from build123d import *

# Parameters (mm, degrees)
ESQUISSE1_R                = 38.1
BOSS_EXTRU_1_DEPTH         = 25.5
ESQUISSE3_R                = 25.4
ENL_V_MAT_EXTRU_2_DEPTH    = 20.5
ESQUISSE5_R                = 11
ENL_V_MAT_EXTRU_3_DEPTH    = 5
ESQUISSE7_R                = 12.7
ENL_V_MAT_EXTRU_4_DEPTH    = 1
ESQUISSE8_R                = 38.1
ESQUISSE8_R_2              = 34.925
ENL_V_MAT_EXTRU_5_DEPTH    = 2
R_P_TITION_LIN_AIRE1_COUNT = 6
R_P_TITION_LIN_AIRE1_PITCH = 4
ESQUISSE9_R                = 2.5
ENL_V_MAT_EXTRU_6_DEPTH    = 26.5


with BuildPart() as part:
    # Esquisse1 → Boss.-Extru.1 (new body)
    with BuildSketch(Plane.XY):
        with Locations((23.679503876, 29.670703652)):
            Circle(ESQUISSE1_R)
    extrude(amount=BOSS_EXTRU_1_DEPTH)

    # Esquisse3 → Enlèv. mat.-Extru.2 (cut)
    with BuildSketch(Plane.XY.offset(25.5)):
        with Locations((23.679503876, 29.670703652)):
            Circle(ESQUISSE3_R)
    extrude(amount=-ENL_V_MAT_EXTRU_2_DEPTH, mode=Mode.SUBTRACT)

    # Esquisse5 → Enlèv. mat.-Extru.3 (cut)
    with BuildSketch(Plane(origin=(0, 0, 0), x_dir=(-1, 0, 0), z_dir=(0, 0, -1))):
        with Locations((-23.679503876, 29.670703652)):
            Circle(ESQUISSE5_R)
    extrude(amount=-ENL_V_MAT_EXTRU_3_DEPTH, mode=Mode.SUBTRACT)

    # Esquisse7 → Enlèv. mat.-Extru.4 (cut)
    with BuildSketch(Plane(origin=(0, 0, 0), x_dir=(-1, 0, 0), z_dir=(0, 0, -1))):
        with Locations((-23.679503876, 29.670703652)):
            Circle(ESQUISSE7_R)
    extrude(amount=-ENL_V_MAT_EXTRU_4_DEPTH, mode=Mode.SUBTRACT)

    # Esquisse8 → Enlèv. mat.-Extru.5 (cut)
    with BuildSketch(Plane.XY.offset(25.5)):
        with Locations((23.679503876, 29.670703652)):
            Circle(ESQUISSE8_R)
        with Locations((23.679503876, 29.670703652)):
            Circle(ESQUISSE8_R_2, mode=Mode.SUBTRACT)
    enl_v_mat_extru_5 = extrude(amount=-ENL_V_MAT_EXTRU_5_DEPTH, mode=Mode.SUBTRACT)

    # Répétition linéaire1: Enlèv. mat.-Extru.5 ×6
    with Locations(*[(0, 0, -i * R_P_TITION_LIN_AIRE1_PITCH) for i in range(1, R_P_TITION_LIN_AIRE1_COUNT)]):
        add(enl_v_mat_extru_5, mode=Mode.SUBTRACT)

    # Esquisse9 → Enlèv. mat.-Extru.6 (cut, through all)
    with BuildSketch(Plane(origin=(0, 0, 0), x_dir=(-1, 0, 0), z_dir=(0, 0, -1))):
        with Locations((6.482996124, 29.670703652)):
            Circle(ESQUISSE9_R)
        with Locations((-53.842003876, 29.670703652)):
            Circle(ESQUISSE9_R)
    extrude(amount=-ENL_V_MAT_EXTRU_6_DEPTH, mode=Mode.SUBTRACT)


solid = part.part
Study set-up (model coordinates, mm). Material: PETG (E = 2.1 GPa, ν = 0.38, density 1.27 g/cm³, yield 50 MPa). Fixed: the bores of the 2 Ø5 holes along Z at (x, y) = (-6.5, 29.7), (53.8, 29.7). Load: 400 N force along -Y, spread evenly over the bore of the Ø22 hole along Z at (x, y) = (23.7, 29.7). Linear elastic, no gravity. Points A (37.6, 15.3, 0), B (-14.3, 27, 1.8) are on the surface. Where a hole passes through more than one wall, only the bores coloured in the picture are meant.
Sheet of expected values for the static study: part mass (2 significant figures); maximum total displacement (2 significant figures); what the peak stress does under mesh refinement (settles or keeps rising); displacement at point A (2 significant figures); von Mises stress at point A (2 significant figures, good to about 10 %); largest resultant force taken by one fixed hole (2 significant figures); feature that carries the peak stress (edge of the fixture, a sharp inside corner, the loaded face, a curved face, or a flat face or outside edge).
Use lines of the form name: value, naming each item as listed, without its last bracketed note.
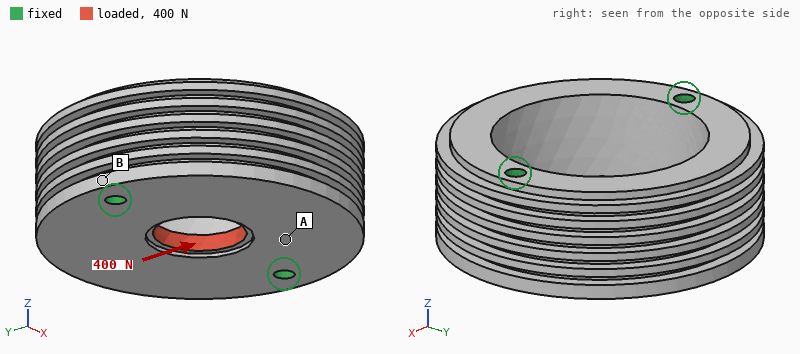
part mass: 80 g
maximum total displacement: 28 µm
what the peak stress does under mesh refinement: keeps rising
displacement at point A: 18 µm
von Mises stress at point A: 0.88 MPa
largest resultant force taken by one fixed hole: 200 N
feature that carries the peak stress: edge of the fixture
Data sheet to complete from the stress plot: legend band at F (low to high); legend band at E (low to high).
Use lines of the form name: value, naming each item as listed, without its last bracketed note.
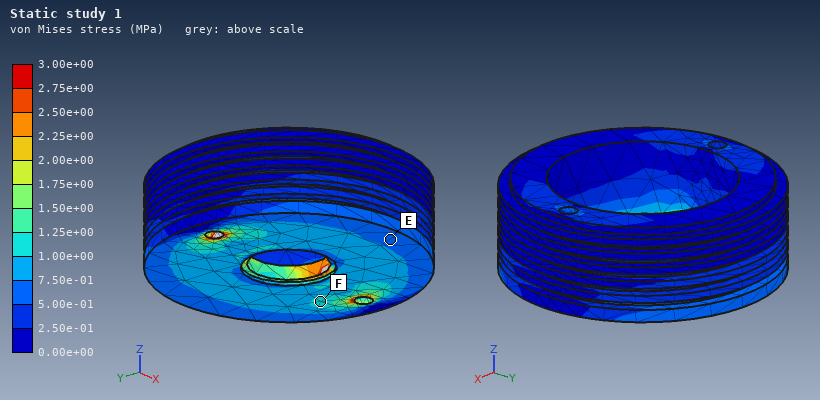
legend band at F: 1.00e+00 to 1.25e+00 MPa
legend band at E: 5.00e-01 to 7.50e-01 MPa
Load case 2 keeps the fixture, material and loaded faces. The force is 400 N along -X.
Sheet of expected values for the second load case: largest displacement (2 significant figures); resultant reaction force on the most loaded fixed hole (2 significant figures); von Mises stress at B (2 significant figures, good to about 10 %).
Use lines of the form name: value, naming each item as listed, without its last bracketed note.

largest displacement: 21 µm
resultant reaction force on the most loaded fixed hole: 200 N
von Mises stress at B: 0.91 MPa
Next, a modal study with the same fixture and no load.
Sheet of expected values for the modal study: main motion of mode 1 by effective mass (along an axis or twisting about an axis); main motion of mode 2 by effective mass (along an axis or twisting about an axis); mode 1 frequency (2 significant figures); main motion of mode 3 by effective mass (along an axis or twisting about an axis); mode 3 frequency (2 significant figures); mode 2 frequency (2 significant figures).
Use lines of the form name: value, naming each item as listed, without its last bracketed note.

main motion of mode 1 by effective mass: twisting about X
main motion of mode 2 by effective mass: along Z
mode 1 frequency: 2100 Hz
main motion of mode 3 by effective mass: twisting about Z
mode 3 frequency: 2900 Hz
mode 2 frequency: 2300 Hz
